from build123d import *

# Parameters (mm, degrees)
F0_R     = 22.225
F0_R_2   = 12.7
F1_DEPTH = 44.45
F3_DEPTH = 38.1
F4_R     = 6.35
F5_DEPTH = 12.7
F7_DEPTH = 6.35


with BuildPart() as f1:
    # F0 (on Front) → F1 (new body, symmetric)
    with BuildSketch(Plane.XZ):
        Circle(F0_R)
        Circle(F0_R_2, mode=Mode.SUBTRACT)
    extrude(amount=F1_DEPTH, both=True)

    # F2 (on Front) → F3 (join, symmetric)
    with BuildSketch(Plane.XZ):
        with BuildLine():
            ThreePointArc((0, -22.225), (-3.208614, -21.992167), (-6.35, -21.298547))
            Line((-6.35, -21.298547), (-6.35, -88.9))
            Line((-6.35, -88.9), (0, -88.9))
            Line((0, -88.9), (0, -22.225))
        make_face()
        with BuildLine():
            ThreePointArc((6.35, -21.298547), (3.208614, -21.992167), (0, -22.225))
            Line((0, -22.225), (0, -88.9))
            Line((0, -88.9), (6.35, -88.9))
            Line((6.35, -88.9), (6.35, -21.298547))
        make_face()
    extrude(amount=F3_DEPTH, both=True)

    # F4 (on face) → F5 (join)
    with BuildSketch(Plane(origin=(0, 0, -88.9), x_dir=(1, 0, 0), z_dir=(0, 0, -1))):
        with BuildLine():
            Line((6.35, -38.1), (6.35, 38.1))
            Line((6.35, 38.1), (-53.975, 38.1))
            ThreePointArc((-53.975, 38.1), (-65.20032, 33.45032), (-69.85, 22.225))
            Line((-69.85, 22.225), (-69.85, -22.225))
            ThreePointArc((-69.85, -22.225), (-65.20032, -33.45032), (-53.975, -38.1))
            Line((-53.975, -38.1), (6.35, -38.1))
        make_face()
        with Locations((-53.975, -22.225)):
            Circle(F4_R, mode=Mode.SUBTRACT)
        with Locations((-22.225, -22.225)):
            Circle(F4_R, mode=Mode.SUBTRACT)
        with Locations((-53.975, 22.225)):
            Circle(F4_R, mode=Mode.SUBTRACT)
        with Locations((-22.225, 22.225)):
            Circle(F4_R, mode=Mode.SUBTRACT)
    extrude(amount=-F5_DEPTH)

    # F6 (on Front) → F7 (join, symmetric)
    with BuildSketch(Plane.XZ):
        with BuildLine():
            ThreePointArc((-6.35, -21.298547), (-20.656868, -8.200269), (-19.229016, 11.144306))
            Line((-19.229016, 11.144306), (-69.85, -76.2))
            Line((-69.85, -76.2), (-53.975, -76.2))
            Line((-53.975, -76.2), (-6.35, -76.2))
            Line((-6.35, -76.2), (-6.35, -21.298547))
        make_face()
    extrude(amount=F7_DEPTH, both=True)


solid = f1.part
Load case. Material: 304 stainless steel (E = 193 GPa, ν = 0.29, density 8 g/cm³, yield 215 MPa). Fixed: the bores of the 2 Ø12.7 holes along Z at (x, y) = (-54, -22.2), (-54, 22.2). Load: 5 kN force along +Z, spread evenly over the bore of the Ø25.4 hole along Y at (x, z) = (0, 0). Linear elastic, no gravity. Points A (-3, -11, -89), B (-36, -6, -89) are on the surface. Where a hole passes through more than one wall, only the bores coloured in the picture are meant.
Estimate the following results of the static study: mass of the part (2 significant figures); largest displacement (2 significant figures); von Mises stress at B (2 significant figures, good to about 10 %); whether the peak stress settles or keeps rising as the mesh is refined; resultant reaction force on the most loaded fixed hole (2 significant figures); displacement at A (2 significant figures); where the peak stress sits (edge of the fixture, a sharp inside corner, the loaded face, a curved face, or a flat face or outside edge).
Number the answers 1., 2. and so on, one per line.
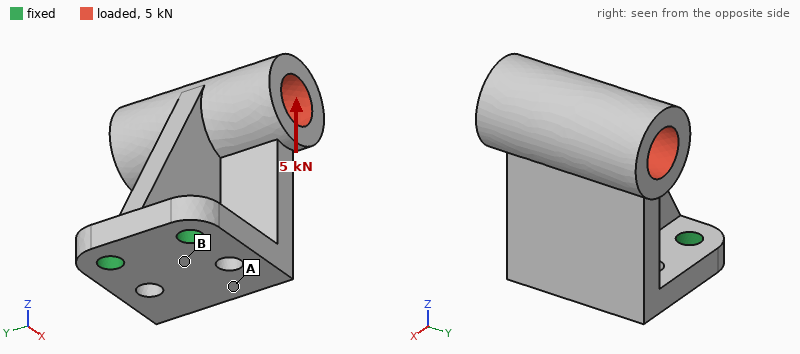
1. 2.0 kg
2. 0.12 mm
3. 35 MPa
4. keeps rising
5. 2.6 kN
6. 0.048 mm
7. edge of the fixture
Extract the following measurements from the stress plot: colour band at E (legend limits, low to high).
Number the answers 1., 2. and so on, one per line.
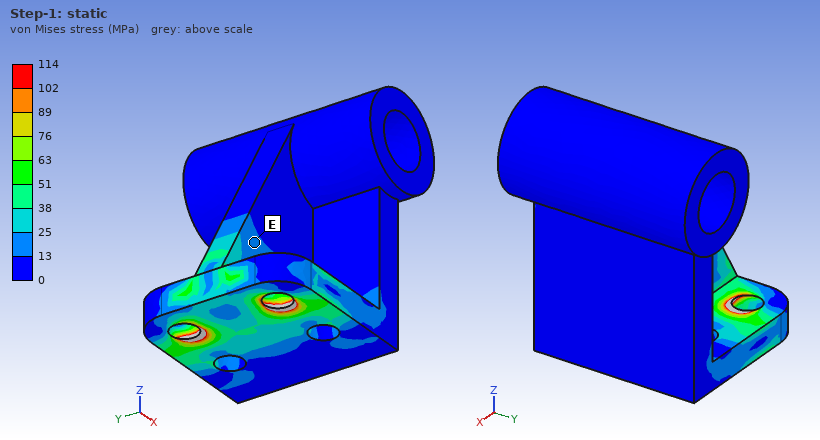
1. 13 to 25 MPa
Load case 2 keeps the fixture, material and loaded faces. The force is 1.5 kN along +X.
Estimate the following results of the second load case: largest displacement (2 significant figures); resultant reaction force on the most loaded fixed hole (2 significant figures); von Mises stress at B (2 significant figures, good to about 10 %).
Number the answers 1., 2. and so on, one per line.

1. 62 µm
2. 750 N
3. 16 MPa
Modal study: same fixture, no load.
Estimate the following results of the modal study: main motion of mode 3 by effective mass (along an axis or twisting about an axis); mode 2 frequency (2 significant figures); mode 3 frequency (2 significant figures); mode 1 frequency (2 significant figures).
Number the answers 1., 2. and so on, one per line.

1. twisting about Z
2. 820 Hz
3. 2200 Hz
4. 800 Hz
